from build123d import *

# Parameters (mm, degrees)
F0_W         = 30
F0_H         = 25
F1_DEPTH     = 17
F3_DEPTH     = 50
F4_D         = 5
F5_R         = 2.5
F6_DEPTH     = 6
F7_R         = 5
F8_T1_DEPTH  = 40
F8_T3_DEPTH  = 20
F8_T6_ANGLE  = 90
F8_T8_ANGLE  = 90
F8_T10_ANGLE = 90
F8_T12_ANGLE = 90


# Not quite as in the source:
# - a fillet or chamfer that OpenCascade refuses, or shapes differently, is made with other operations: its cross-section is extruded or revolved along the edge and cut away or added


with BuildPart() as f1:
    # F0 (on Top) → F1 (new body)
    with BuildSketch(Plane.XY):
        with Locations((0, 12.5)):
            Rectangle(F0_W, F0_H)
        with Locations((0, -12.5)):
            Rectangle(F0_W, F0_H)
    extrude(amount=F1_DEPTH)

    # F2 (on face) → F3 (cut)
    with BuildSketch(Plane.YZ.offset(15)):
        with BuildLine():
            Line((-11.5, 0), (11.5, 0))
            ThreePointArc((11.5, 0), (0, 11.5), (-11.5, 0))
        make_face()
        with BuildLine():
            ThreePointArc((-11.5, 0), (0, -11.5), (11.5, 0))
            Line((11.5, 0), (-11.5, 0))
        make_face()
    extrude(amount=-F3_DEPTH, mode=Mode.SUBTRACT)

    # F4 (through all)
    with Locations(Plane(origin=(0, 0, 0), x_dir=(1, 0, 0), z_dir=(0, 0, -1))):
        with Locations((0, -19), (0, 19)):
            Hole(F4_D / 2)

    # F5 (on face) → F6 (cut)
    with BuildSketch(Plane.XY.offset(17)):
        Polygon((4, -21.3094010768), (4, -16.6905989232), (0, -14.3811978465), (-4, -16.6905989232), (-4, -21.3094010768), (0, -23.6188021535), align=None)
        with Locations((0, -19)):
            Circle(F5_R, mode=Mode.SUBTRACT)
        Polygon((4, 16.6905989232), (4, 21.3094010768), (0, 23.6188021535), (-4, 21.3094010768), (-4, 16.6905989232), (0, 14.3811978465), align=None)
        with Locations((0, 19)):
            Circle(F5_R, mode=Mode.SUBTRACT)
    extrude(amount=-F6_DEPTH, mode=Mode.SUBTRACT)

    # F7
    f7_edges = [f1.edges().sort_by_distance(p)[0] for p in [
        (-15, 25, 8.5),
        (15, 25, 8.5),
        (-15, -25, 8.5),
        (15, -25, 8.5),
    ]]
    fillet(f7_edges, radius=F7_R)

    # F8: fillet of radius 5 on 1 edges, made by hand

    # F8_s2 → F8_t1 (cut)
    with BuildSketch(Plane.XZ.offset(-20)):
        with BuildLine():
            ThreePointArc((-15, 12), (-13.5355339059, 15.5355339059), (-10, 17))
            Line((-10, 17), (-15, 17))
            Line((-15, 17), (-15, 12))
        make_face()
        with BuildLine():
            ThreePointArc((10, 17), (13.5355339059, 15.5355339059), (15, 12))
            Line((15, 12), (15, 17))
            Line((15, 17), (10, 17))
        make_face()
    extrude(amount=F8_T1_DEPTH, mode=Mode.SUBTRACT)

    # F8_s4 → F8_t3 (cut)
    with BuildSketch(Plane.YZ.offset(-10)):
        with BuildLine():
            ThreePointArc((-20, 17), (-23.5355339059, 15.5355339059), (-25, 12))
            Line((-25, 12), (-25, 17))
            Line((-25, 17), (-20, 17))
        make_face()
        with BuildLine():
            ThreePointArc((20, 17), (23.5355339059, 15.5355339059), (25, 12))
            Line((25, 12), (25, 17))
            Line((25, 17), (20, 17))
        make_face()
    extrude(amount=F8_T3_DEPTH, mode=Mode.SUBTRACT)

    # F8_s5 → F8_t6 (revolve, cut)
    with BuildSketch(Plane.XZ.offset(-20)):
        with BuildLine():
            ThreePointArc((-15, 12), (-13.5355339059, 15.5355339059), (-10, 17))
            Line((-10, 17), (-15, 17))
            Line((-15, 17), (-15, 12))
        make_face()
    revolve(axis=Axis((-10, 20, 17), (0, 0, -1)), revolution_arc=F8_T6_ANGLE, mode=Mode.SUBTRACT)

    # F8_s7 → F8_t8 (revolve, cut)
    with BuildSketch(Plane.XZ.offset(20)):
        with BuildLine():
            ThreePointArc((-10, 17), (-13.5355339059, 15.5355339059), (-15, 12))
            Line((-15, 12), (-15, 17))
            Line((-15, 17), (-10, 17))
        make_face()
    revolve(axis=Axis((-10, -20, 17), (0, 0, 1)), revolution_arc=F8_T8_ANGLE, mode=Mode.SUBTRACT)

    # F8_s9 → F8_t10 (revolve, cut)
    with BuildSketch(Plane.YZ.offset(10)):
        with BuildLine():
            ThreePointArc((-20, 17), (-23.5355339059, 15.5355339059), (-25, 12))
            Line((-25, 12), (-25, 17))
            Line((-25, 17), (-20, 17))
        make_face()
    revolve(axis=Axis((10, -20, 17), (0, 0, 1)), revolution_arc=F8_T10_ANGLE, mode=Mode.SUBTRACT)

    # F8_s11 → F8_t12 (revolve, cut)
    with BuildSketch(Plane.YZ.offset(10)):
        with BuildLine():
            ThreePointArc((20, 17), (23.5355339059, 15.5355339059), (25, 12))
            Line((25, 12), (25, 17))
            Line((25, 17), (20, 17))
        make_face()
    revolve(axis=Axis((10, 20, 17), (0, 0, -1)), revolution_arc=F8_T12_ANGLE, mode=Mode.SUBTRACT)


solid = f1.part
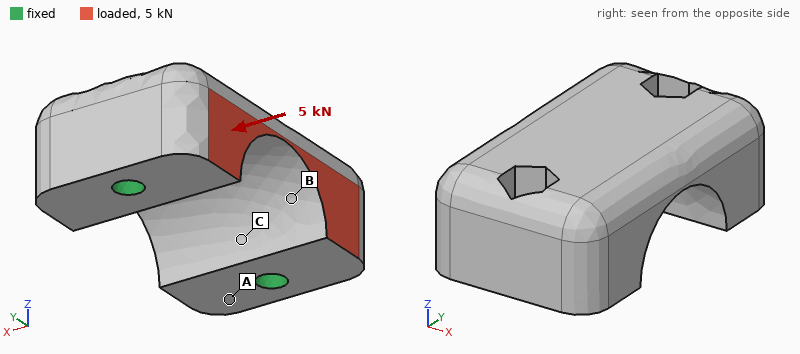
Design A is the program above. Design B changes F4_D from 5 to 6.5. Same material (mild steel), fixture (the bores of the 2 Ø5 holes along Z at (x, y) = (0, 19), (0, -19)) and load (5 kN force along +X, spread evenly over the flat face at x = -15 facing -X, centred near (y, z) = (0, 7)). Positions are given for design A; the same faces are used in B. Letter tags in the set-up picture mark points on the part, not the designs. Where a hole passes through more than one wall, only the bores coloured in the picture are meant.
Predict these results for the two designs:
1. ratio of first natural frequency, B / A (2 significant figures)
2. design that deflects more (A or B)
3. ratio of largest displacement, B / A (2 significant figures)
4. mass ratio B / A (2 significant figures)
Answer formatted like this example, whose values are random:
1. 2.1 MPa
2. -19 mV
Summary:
1. 1.2
2. A
3. 0.89
4. 0.98
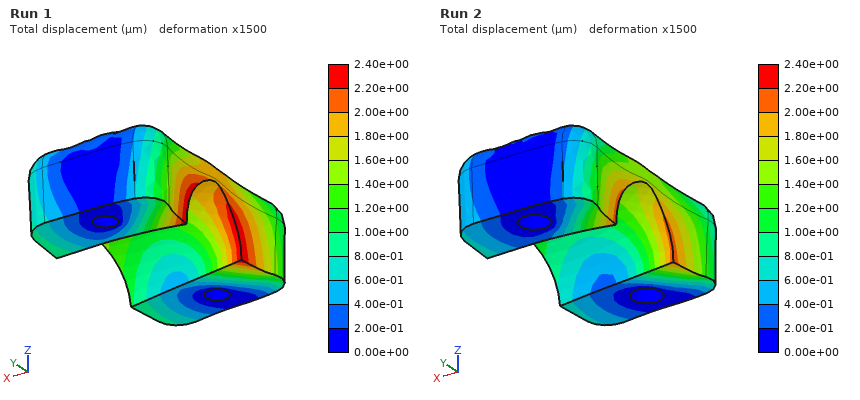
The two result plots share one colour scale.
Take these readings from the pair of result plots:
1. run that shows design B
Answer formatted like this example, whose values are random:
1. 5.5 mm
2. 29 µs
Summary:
1. Run 2
